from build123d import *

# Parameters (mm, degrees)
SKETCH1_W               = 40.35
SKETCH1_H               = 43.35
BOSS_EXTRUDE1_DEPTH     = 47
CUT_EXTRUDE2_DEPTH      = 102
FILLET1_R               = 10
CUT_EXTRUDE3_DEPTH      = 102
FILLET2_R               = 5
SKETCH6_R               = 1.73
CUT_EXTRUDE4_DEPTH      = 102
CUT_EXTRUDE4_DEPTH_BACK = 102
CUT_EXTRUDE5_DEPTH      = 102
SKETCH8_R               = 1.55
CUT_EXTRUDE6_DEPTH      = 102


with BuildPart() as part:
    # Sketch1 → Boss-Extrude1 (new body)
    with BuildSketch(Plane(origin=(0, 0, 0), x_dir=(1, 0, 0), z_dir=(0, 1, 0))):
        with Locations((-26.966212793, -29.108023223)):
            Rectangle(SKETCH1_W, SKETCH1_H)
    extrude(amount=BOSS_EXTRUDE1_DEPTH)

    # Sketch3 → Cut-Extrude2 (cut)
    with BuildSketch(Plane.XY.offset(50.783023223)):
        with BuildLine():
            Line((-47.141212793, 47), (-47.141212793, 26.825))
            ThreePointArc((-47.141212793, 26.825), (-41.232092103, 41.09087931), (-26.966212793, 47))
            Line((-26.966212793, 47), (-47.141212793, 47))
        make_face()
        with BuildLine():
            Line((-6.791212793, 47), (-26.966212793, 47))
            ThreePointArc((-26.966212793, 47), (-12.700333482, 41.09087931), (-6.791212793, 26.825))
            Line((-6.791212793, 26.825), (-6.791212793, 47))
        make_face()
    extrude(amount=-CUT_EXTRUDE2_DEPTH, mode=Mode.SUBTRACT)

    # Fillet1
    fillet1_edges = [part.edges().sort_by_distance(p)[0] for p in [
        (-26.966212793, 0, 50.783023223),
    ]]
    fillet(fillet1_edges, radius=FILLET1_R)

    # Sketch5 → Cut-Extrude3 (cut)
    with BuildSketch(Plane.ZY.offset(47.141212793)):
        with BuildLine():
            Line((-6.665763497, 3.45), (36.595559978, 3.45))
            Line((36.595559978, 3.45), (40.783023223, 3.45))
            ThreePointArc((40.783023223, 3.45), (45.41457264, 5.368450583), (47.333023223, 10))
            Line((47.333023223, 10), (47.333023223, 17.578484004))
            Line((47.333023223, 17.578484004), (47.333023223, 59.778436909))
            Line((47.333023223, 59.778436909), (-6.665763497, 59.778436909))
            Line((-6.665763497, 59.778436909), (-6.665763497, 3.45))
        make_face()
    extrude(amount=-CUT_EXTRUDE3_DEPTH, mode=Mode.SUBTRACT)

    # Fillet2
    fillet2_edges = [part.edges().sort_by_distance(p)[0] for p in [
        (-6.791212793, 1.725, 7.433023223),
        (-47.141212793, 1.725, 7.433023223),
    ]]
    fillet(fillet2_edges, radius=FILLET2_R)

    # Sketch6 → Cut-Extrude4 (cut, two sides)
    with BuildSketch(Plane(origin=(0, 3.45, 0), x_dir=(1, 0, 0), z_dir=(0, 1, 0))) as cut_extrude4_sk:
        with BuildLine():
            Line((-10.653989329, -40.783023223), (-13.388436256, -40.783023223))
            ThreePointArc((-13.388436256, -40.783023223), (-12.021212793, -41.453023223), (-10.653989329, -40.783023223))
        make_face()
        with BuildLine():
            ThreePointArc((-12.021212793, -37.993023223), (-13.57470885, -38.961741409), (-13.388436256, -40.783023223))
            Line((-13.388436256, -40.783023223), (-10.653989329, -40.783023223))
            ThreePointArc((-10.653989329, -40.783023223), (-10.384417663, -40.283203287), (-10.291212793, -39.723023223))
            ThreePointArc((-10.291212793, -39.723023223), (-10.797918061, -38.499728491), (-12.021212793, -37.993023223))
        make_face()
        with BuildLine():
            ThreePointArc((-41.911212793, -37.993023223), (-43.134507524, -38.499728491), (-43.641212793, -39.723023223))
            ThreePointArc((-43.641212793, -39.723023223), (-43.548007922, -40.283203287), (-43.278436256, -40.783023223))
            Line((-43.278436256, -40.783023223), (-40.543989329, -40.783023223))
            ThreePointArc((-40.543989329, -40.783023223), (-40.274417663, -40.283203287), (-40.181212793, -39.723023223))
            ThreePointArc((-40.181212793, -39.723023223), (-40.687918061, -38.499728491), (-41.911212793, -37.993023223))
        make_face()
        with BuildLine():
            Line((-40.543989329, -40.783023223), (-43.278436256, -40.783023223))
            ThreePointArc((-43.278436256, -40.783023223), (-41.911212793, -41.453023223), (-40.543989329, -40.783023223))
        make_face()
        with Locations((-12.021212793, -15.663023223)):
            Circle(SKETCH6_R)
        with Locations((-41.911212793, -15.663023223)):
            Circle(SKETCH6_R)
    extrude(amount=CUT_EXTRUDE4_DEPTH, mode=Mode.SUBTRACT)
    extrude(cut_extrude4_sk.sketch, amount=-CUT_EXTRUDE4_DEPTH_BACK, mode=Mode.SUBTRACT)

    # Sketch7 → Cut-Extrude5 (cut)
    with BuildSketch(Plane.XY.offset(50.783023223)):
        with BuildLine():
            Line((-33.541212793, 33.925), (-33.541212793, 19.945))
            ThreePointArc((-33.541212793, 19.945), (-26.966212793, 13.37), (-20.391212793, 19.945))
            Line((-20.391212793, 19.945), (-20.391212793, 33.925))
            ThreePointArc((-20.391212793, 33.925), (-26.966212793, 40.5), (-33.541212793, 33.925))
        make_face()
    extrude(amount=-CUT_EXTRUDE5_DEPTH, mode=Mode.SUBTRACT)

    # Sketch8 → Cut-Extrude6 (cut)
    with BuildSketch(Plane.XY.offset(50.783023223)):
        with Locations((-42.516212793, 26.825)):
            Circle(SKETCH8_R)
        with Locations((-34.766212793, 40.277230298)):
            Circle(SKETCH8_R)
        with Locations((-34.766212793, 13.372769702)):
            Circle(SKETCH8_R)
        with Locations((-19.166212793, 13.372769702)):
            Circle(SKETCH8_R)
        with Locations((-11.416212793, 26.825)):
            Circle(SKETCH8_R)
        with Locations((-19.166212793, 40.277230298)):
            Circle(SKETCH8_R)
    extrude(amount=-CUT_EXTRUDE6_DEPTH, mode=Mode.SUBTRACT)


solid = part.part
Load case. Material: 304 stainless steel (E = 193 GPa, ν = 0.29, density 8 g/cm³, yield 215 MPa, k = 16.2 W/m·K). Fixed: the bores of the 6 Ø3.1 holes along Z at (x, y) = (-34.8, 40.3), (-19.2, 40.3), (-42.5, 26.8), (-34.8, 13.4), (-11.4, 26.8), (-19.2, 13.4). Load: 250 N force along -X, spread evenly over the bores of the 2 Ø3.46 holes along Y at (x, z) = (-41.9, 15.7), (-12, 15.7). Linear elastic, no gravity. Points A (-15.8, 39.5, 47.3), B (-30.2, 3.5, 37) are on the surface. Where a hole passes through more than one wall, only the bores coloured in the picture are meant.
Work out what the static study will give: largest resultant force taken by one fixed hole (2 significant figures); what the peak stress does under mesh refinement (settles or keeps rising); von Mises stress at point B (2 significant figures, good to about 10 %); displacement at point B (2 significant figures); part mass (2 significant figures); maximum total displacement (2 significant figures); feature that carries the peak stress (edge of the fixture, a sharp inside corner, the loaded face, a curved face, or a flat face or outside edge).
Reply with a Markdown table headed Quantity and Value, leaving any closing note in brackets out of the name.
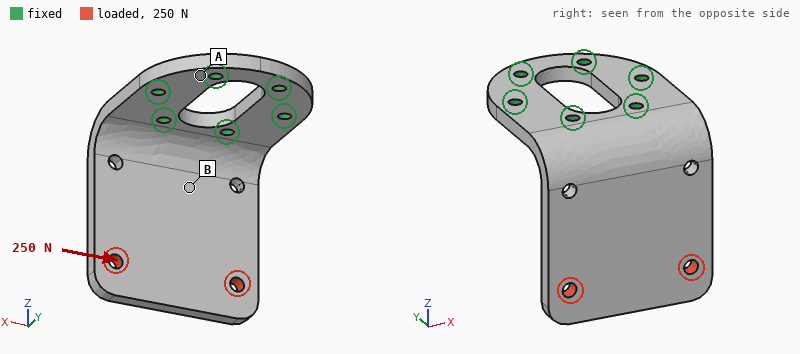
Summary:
| Quantity | Value |
|---|---|
| largest resultant force taken by one fixed hole | 460 N |
| what the peak stress does under mesh refinement | keeps rising |
| von Mises stress at point B | 16 MPa |
| displacement at point B | 10 µm |
| part mass | 77 g |
| maximum total displacement | 41 µm |
| feature that carries the peak stress | edge of the fixture |
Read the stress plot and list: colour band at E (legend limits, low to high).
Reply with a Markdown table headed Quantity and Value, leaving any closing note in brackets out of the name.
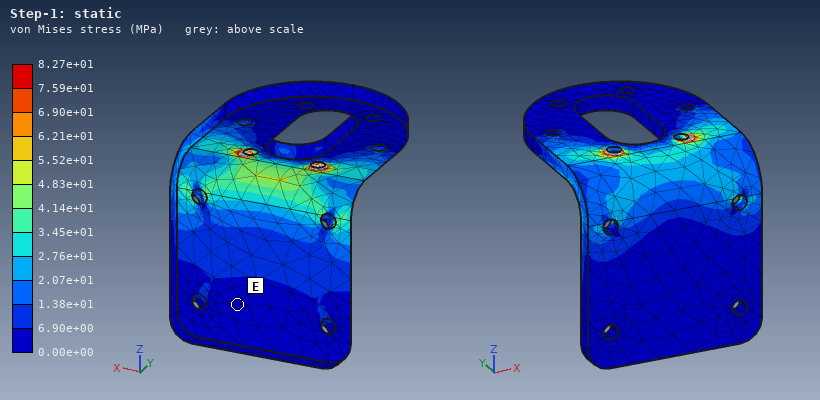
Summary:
| Quantity | Value |
|---|---|
| colour band at E | 0.00e+00 to 6.90e+00 MPa |
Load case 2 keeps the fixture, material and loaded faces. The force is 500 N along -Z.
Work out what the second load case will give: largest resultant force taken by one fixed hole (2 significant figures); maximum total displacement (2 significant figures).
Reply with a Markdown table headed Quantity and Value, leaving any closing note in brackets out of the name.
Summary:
| Quantity | Value |
|---|---|
| largest resultant force taken by one fixed hole | 300 N |
| maximum total displacement | 64 µm |
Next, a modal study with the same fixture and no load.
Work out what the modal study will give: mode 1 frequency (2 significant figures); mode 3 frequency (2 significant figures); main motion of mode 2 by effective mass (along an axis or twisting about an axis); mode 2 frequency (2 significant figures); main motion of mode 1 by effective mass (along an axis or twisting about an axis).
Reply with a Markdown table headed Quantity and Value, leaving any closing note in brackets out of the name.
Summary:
| Quantity | Value |
|---|---|
| mode 1 frequency | 1200 Hz |
| mode 3 frequency | 4300 Hz |
| main motion of mode 2 by effective mass | along X |
| mode 2 frequency | 2600 Hz |
| main motion of mode 1 by effective mass | along Y |
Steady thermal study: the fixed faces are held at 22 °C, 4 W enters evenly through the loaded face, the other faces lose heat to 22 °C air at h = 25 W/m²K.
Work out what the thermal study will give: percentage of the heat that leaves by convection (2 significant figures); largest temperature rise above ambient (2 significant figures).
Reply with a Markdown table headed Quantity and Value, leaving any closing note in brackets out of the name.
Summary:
| Quantity | Value |
|---|---|
| percentage of the heat that leaves by convection | 62 % |
| largest temperature rise above ambient | 49 K |
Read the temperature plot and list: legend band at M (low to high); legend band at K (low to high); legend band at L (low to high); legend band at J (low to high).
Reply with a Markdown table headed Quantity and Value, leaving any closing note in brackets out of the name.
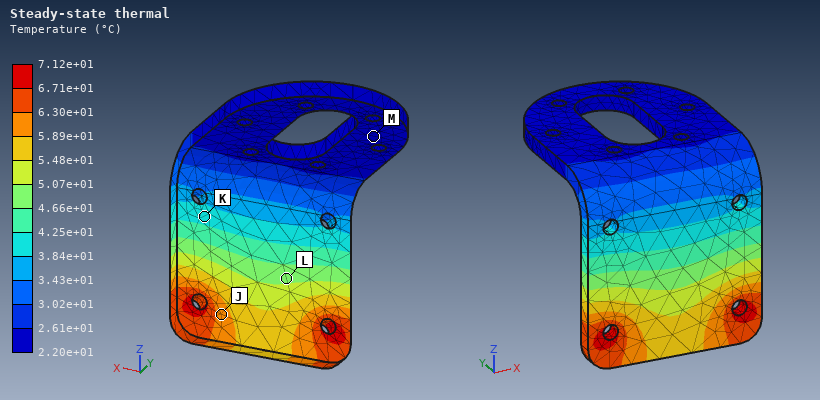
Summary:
| Quantity | Value |
|---|---|
| legend band at M | 2.20e+01 to 2.61e+01 °C |
| legend band at K | 3.84e+01 to 4.25e+01 °C |
| legend band at L | 4.66e+01 to 5.07e+01 °C |
| legend band at J | 5.89e+01 to 6.30e+01 °C |
